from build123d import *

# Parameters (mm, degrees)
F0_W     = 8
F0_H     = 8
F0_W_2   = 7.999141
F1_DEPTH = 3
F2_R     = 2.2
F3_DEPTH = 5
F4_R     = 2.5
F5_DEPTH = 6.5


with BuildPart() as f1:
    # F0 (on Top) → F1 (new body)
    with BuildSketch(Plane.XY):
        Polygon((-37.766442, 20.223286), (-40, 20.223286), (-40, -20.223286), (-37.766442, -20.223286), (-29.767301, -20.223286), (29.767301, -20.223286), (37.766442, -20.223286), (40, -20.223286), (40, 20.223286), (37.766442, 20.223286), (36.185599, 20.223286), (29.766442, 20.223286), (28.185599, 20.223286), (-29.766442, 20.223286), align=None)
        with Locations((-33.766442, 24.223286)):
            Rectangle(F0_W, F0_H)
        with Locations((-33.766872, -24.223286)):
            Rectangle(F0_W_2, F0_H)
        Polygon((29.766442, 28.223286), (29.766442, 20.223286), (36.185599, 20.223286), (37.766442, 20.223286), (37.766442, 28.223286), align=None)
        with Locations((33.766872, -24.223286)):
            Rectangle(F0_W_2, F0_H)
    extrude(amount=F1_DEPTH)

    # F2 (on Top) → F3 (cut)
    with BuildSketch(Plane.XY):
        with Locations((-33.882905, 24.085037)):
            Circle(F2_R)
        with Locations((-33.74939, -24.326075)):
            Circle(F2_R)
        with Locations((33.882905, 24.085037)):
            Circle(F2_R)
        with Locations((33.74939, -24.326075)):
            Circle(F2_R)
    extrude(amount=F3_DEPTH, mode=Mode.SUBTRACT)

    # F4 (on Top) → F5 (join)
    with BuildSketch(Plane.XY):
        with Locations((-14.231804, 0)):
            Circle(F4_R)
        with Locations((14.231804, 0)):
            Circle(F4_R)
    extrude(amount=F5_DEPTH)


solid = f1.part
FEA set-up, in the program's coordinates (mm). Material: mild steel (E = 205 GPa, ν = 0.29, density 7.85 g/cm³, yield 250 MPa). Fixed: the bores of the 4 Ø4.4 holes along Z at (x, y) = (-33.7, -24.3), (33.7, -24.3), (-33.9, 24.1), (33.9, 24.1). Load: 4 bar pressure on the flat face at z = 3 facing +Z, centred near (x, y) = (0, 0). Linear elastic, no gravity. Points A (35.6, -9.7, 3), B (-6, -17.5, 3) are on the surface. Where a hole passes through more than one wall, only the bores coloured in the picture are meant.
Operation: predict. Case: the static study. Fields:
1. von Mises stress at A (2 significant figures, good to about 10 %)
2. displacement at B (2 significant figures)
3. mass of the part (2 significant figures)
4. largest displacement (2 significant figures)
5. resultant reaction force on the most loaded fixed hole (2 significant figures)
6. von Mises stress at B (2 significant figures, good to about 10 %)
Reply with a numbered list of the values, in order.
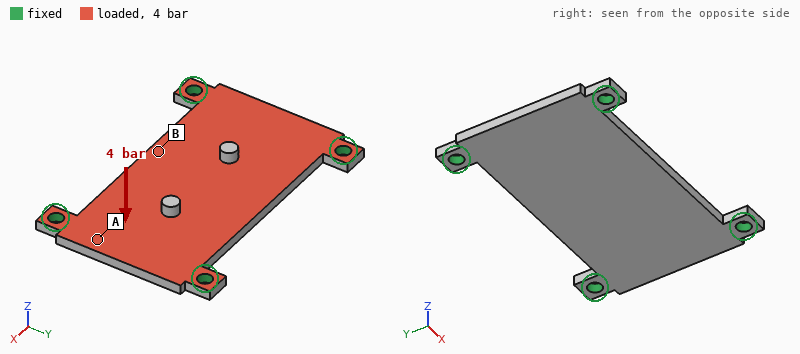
1. 33 MPa
2. 86 µm
3. 82 g
4. 93 µm
5. 340 N
6. 70 MPa
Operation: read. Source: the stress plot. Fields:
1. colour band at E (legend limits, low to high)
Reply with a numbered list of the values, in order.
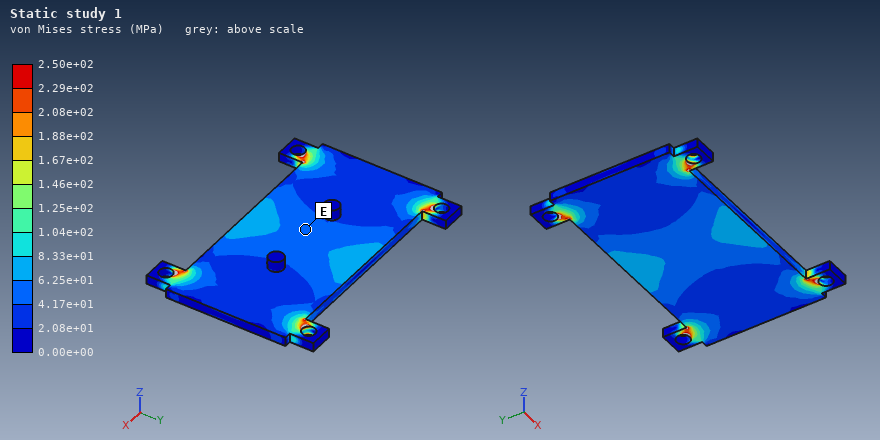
1. 4.17e+01 to 6.25e+01 MPa
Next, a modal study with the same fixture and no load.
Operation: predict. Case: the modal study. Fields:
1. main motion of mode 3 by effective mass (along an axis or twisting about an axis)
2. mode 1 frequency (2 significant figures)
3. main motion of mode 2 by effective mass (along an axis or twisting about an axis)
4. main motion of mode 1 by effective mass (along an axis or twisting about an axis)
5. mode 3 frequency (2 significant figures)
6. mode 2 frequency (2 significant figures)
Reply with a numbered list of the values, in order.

1. twisting about Y
2. 2400 Hz
3. twisting about X
4. along Z
5. 5900 Hz
6. 4800 Hz
